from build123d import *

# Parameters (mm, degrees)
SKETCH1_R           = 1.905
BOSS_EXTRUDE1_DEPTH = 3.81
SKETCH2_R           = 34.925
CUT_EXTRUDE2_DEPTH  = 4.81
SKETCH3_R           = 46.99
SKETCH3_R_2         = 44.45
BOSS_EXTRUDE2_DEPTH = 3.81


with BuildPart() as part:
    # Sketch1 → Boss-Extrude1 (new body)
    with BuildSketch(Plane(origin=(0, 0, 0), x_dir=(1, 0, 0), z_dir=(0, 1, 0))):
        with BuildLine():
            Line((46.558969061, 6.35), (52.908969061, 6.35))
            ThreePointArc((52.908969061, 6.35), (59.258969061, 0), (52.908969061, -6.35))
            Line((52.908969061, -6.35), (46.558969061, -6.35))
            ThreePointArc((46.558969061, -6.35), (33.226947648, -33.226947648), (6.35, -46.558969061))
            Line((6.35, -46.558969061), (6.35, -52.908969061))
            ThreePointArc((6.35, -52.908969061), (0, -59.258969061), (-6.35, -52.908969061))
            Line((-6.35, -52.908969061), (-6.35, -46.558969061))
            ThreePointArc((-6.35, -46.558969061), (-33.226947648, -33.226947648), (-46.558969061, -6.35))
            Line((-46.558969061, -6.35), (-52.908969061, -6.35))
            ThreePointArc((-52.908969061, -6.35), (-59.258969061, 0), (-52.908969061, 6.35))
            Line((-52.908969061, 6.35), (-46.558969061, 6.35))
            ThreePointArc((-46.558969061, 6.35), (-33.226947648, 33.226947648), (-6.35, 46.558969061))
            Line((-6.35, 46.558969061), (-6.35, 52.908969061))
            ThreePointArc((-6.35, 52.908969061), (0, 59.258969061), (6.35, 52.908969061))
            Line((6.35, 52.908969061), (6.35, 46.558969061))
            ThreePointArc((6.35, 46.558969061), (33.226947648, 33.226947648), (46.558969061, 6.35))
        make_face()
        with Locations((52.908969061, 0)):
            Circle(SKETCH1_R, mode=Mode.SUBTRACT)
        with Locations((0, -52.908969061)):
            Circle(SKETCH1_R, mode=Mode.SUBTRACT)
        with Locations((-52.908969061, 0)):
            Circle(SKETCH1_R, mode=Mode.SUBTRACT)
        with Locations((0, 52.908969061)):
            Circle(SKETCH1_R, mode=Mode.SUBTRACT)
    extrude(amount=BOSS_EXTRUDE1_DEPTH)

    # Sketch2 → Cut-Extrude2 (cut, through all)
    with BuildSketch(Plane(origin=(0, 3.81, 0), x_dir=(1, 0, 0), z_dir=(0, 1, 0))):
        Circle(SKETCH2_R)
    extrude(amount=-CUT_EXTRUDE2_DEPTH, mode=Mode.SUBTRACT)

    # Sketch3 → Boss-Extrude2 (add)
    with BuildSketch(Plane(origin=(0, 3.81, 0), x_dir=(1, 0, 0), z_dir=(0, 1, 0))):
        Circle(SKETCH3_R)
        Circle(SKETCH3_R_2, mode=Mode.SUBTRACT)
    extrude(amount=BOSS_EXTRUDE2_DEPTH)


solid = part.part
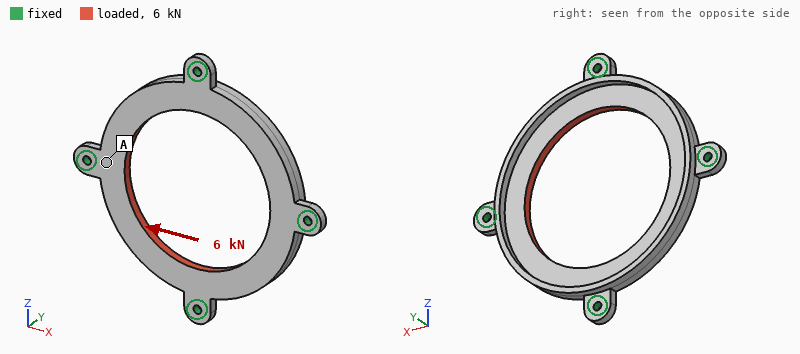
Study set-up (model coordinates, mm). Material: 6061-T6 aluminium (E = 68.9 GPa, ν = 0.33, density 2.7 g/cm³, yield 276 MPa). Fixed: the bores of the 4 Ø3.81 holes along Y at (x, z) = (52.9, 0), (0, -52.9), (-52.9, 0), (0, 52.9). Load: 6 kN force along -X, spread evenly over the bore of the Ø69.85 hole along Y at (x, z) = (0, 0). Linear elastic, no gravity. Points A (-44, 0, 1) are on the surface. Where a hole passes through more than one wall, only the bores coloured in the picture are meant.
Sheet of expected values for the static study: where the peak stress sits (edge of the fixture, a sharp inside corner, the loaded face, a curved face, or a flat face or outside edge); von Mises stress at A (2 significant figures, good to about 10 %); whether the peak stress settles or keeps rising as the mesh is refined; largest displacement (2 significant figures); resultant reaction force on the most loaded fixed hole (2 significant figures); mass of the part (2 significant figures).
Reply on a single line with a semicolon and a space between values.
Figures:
edge of the fixture; 17 MPa; keeps rising; 45 µm; 1.7 kN; 45 g
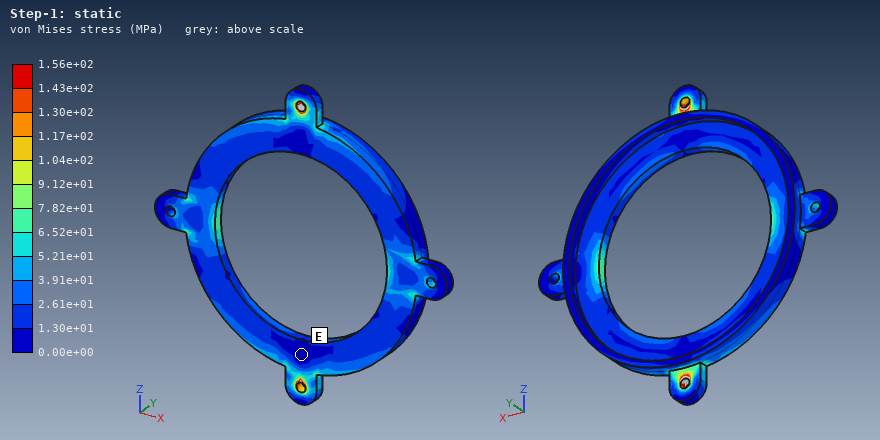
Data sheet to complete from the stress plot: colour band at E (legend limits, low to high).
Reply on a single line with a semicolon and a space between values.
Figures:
0.00e+00 to 1.30e+01 MPa
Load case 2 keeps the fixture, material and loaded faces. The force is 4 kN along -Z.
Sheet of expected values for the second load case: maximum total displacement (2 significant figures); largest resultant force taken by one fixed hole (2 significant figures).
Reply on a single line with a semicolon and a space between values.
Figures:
30 µm; 1.1 kN
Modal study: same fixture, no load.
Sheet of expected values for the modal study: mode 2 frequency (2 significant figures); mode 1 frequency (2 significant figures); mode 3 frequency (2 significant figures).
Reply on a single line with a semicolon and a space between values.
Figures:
4200 Hz; 3600 Hz; 4200 Hz
